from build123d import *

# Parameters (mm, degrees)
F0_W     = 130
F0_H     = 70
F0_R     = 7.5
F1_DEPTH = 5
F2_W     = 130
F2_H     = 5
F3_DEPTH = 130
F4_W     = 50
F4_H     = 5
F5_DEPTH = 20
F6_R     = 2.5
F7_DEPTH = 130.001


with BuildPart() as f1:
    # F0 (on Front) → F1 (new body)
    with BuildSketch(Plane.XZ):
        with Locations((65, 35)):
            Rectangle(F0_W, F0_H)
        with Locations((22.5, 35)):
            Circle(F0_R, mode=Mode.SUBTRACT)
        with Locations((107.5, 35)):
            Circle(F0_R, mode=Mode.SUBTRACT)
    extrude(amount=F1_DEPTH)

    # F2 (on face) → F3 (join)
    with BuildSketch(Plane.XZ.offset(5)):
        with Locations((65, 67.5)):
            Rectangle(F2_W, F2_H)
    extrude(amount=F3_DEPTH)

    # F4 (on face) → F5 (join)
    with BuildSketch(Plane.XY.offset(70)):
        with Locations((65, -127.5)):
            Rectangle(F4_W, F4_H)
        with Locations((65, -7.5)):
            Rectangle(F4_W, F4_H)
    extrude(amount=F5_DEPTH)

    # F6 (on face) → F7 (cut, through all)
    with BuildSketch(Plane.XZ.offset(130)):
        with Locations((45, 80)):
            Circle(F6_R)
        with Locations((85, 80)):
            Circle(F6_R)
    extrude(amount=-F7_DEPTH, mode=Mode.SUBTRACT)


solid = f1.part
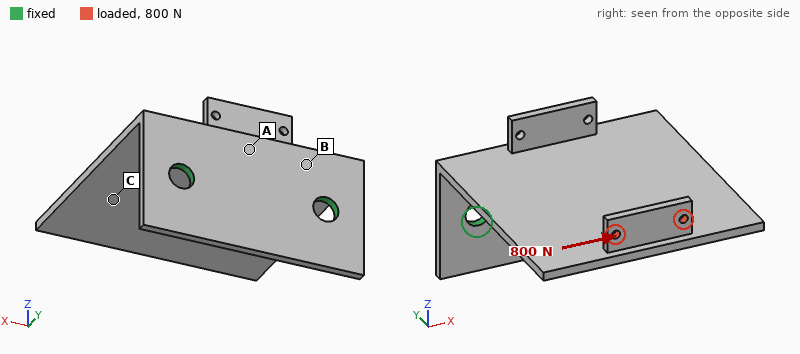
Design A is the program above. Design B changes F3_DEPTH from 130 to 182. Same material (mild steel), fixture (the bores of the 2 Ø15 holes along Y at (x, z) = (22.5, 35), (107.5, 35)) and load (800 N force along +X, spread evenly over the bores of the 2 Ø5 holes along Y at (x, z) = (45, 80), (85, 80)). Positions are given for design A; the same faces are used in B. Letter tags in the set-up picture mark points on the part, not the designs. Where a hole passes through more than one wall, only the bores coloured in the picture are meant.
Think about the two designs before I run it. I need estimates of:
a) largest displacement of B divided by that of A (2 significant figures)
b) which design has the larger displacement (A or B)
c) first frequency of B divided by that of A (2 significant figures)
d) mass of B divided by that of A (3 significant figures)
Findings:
1.3
B
0.59
1.25
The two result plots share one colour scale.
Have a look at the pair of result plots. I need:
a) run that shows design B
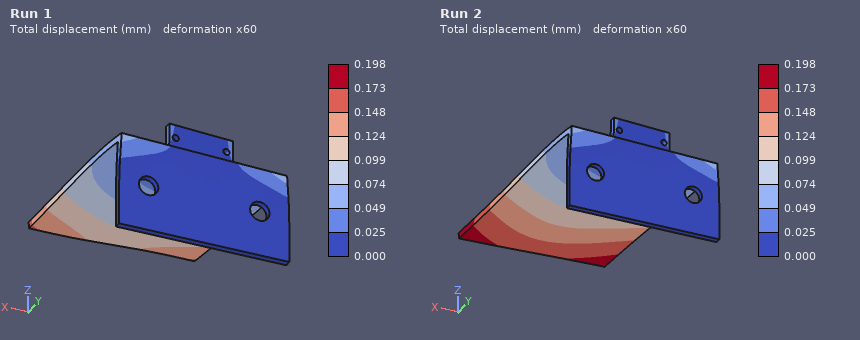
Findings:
Run 2
